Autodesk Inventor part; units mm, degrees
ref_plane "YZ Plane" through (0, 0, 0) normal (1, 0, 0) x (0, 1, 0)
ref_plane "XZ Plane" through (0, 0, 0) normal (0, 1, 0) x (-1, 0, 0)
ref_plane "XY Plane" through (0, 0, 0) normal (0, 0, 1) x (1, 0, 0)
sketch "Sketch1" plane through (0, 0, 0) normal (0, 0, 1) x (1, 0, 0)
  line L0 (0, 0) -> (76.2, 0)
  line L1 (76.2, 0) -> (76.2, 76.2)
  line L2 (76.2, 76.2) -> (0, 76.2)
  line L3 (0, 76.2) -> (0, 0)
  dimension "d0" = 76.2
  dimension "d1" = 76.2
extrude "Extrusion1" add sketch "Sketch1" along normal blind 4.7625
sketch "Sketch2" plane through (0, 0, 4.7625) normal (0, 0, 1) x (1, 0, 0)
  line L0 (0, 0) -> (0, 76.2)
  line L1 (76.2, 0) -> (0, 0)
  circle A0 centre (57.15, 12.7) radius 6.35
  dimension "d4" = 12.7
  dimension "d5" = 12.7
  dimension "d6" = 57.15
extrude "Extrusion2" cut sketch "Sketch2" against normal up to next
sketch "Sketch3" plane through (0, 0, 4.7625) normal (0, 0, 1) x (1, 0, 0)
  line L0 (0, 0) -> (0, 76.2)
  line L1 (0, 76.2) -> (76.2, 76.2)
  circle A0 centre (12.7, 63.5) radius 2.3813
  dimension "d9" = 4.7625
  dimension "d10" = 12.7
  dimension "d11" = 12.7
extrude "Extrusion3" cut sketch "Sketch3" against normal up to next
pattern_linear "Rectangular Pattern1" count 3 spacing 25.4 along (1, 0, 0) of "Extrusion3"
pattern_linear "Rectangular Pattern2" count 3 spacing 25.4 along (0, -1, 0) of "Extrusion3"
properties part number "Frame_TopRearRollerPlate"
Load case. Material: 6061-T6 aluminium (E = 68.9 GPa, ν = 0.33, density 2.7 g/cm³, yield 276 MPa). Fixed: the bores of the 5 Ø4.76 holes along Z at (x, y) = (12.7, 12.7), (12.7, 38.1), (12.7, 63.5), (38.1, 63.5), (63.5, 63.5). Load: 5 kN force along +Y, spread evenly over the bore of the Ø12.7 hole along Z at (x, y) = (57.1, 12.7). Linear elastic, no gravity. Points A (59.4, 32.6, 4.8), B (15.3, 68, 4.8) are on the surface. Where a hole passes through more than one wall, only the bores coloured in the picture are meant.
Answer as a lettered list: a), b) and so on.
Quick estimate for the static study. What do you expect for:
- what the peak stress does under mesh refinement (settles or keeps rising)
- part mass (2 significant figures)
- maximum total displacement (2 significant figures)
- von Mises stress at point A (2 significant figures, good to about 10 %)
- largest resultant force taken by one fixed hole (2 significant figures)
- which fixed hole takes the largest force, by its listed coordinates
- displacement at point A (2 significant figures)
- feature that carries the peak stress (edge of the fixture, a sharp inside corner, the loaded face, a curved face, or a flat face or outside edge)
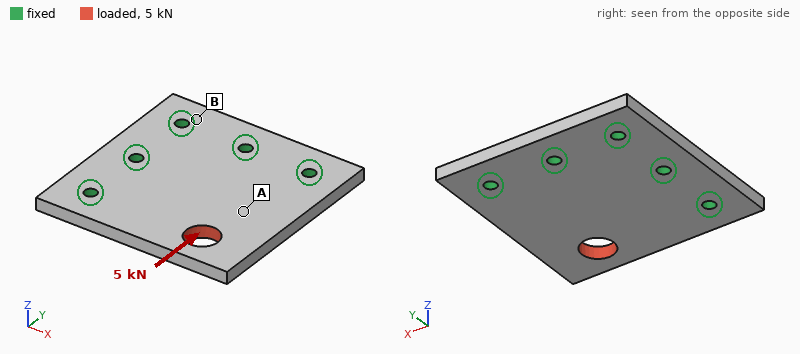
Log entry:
a) keeps rising
b) 72 g
c) 32 µm
d) 27 MPa
e) 2.7 kN
f) (63.5, 63.5)
g) 12 µm
h) edge of the fixture
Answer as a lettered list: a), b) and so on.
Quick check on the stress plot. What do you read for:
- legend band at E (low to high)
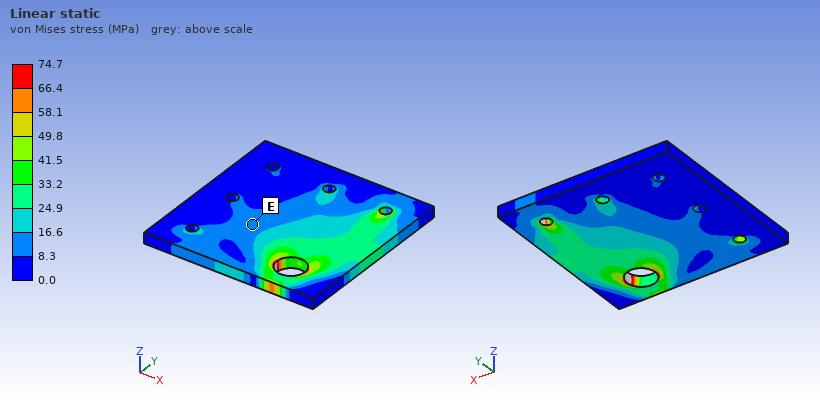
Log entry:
a) 8.3 to 16.6 MPa
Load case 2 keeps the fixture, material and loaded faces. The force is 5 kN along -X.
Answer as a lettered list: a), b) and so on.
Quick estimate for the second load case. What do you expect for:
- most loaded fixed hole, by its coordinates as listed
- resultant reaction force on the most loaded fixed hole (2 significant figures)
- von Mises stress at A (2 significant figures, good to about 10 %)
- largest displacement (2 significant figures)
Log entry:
a) (12.7, 12.7)
b) 3.1 kN
c) 12 MPa
d) 31 µm
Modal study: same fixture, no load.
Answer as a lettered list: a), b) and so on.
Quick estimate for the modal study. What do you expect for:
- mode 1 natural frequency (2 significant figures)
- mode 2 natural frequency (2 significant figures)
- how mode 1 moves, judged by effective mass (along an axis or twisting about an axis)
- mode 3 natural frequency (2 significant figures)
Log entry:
a) 2000 Hz
b) 6100 Hz
c) along Z
d) 6900 Hz
